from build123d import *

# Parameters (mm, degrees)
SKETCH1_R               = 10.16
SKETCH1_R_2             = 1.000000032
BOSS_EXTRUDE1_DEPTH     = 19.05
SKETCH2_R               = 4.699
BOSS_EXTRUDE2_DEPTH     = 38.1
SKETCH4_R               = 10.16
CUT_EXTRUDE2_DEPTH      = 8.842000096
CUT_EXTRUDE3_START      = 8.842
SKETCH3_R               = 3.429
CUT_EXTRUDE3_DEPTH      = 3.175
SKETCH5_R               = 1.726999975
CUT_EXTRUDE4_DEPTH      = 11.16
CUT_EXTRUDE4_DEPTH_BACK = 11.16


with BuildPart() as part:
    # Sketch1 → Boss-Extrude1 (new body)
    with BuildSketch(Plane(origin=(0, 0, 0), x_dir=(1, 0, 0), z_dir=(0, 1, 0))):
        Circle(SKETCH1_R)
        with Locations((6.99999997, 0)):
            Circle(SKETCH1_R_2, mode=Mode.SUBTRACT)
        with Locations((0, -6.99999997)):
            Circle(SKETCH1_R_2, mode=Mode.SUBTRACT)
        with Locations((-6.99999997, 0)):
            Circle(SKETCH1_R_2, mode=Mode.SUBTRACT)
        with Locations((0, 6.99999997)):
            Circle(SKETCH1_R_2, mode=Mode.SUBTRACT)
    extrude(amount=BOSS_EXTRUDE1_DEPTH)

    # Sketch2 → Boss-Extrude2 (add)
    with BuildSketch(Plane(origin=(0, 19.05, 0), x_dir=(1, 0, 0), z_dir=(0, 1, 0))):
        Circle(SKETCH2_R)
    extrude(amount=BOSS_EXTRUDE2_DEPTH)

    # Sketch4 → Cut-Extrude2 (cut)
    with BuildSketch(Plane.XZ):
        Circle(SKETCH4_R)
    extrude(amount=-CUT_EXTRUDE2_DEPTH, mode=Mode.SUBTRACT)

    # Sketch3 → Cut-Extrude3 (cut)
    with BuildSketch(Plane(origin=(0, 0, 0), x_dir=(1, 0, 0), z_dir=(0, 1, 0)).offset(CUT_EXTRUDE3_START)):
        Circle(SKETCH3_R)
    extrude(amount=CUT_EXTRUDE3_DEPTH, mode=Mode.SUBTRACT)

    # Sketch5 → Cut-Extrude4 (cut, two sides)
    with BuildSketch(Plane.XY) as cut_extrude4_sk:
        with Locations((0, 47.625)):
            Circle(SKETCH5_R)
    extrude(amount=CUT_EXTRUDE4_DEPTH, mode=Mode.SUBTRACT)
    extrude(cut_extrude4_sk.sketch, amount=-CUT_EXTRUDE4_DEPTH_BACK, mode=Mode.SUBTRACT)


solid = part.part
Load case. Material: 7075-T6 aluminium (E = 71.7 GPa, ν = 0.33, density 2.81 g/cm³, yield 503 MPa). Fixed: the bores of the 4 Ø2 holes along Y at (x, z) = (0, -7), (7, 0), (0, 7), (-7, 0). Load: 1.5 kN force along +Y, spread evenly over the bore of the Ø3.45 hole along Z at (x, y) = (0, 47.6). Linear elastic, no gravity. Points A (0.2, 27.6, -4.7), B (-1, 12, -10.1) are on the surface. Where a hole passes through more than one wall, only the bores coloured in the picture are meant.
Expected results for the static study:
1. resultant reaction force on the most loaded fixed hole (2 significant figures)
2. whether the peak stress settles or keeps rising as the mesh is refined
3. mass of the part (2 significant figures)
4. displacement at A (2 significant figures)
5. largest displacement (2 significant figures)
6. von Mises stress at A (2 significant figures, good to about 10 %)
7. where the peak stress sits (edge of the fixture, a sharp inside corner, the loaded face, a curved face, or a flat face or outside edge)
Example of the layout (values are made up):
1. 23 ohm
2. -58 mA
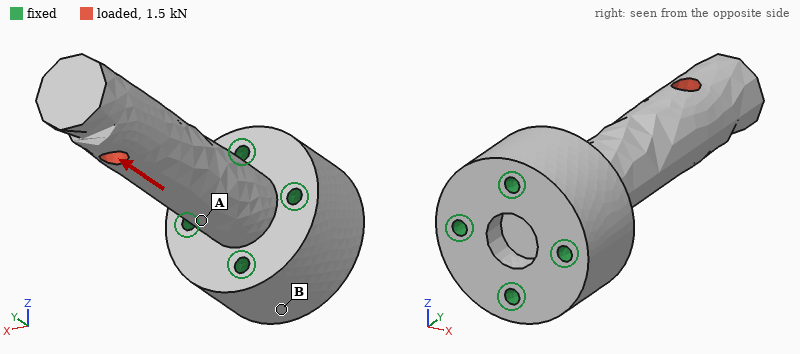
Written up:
1. 410 N
2. keeps rising
3. 16 g
4. 3.8 µm
5. 11 µm
6. 21 MPa
7. a sharp inside corner
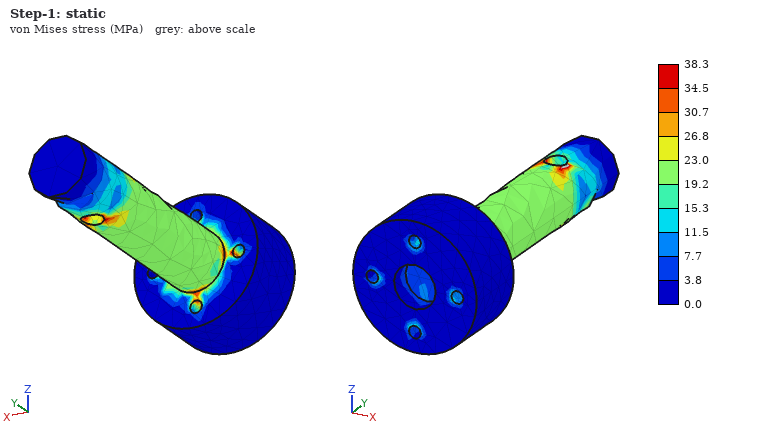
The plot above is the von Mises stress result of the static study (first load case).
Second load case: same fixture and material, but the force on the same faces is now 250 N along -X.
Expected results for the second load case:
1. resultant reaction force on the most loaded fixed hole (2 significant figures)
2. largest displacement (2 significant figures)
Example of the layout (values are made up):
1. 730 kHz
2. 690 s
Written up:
1. 530 N
2. 0.13 mm
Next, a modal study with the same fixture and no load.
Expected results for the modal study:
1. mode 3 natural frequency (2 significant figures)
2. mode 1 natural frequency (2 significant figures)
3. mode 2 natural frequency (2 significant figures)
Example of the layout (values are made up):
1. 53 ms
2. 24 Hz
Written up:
1. 20 kHz
2. 4100 Hz
3. 4200 Hz
